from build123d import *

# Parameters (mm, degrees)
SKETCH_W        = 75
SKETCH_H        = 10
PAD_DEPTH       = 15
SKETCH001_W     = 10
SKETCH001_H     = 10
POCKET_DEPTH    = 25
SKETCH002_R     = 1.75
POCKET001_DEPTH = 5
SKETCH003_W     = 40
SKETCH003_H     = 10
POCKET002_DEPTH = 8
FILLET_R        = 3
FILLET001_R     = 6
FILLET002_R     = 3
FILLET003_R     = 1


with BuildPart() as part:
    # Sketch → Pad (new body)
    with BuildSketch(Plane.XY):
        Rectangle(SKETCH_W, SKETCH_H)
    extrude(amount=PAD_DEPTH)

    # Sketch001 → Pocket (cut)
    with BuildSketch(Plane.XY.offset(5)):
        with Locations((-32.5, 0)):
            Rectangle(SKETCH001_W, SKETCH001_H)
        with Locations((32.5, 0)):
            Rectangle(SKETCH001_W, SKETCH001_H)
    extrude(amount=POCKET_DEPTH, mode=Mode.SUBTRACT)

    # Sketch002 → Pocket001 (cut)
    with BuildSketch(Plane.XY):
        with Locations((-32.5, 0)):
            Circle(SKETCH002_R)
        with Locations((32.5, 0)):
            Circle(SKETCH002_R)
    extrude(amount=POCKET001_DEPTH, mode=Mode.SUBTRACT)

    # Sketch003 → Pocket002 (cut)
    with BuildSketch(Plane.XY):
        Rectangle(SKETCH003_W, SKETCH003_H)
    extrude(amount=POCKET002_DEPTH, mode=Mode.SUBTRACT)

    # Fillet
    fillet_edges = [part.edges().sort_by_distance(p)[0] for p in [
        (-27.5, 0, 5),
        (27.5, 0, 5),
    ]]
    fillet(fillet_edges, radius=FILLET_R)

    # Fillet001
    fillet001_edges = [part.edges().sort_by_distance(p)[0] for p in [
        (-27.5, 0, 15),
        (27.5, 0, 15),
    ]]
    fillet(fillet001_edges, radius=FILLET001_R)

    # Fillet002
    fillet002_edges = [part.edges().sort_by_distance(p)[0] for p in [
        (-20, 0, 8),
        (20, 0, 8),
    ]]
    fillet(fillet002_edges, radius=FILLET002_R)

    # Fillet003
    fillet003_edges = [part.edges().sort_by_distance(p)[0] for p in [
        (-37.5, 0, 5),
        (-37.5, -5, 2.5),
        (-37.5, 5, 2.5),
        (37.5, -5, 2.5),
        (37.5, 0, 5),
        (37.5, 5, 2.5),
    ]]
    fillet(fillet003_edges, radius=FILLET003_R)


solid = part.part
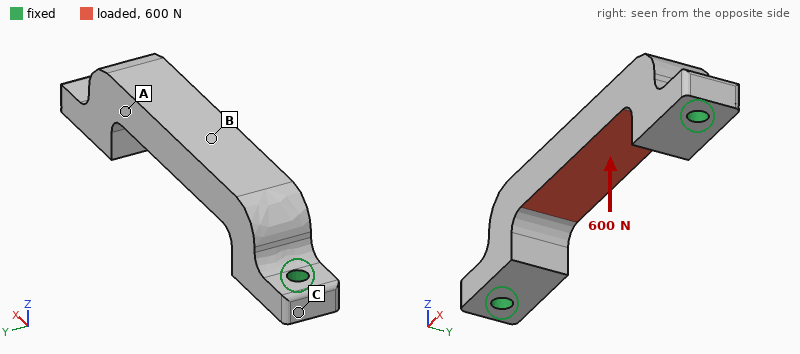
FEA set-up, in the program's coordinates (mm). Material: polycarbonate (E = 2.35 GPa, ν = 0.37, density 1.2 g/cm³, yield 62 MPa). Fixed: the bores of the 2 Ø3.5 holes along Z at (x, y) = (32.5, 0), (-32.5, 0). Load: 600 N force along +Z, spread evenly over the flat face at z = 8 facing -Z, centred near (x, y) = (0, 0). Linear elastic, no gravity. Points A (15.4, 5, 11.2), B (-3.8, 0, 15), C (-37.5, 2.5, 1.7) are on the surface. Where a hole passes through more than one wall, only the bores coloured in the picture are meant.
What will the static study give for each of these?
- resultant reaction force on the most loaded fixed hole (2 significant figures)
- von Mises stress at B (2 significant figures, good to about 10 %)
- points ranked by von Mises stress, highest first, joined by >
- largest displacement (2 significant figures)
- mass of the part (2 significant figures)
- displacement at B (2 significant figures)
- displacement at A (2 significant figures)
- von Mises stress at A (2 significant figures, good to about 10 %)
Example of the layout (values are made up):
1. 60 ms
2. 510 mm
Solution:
1. 560 N
2. 26 MPa
3. B > A > C
4. 0.55 mm
5. 7.0 g
6. 0.51 mm
7. 0.27 mm
8. 14 MPa
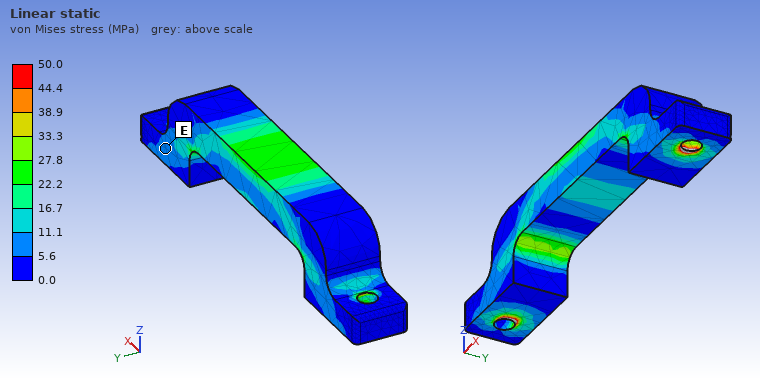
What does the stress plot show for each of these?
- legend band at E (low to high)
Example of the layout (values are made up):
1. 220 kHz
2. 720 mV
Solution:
1. 5.6 to 11.1 MPa
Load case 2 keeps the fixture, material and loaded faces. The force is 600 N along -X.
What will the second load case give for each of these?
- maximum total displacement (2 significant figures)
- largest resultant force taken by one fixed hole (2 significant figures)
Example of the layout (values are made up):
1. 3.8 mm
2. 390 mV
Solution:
1. 0.24 mm
2. 300 N
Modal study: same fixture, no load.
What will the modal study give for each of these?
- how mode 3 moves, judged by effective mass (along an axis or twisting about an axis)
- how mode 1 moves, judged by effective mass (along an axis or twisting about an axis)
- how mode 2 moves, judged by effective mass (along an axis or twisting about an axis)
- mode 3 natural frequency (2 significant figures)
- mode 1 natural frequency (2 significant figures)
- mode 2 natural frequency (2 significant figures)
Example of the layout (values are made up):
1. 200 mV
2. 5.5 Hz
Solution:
1. along X
2. along Y
3. along Z
4. 3700 Hz
5. 1800 Hz
6. 3300 Hz
